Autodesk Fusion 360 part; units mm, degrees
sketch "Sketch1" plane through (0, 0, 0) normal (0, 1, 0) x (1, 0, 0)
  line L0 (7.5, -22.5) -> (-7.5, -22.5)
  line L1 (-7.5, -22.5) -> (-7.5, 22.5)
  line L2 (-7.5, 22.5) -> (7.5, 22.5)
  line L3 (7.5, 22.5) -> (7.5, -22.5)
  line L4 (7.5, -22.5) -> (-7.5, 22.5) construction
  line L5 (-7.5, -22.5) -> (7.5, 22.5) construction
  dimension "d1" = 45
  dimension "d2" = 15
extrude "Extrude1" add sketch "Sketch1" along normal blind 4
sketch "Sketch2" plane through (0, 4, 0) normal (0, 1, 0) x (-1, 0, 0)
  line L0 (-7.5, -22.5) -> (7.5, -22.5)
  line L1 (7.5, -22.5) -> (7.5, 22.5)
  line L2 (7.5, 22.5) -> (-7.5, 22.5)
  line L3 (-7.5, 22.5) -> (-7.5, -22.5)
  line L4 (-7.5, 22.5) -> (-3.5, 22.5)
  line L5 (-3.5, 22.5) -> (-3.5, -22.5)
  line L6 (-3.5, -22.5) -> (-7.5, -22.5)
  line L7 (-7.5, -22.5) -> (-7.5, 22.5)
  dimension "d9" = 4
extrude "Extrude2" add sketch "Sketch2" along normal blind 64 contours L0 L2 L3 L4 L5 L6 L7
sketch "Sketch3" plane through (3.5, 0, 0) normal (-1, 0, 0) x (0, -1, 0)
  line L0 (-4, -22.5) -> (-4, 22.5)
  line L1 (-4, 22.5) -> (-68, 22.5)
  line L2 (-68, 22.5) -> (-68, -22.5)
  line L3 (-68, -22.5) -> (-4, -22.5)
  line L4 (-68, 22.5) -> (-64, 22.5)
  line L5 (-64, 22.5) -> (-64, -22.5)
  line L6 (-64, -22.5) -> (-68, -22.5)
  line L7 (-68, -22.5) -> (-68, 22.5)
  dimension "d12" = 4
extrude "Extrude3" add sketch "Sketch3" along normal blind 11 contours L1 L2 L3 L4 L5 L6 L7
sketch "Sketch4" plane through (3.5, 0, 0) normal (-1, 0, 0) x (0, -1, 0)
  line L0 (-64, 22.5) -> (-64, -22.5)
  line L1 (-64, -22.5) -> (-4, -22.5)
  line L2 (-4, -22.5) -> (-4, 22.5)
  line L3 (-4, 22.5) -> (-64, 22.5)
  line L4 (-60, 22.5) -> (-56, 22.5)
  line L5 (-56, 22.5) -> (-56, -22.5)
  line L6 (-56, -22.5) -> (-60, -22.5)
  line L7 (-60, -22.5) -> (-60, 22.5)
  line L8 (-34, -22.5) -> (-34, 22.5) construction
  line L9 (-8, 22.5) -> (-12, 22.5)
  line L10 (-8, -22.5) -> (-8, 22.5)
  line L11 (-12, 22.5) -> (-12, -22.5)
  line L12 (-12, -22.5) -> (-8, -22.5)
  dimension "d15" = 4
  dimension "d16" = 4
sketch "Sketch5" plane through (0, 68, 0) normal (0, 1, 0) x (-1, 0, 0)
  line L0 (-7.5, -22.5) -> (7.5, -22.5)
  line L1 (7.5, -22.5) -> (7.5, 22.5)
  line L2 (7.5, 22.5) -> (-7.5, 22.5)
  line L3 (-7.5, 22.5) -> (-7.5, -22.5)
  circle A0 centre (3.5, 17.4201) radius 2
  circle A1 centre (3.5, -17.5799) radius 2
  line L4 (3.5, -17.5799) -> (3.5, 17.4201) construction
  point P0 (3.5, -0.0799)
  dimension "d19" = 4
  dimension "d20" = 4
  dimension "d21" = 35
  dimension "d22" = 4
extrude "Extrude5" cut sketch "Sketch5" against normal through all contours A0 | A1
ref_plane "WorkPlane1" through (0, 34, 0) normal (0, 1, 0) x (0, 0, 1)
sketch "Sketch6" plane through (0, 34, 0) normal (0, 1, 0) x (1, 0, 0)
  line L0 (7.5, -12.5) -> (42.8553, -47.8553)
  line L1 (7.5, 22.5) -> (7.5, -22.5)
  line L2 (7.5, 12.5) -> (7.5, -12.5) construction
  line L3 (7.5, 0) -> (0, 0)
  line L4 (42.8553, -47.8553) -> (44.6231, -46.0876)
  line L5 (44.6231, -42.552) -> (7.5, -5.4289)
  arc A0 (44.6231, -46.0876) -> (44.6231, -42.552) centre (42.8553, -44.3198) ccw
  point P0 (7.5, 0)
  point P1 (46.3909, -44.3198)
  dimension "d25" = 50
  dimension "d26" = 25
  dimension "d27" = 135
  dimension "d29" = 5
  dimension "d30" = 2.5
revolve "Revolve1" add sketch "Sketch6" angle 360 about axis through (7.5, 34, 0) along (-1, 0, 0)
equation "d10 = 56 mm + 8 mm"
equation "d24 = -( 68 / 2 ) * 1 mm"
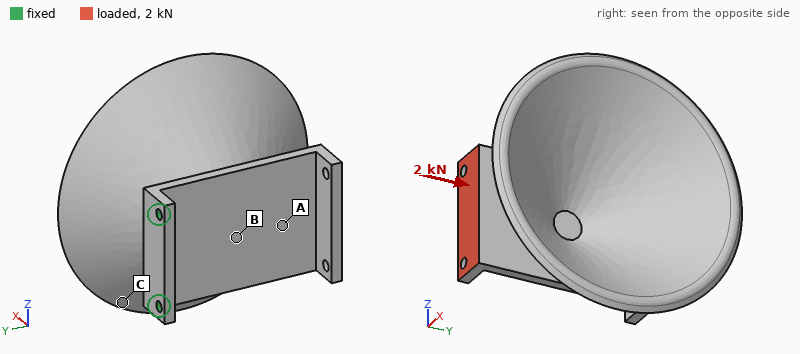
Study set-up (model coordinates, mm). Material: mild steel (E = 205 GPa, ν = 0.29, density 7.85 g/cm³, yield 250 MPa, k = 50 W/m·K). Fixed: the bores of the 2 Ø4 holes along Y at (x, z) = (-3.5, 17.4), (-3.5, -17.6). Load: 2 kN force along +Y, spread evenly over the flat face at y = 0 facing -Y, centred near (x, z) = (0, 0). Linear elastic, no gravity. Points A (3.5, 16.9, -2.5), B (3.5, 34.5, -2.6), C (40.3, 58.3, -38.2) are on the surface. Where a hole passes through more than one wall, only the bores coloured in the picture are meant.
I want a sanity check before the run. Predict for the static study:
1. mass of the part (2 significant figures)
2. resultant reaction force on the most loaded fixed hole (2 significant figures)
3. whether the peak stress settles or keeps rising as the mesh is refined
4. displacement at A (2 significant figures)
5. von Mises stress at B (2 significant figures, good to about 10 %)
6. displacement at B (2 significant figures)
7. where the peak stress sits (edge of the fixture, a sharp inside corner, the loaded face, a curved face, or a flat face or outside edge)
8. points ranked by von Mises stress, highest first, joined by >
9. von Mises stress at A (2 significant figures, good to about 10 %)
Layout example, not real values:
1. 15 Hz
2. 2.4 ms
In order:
1. 480 g
2. 1.0 kN
3. keeps rising
4. 0.20 mm
5. 26 MPa
6. 0.098 mm
7. edge of the fixture
8. A > B > C
9. 98 MPa
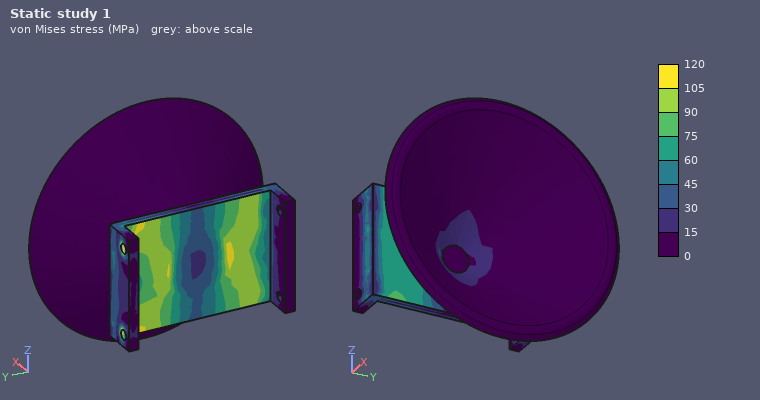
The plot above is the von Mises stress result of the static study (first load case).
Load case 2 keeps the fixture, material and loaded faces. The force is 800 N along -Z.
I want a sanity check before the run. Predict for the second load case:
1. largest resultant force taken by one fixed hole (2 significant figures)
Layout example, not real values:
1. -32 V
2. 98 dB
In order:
1. 1.5 kN
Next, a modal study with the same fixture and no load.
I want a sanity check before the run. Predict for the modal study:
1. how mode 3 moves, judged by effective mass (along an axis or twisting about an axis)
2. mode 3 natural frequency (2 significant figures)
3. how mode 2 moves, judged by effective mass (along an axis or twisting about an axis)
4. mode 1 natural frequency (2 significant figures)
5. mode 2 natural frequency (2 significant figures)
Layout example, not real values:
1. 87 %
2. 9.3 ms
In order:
1. along Z
2. 1300 Hz
3. along Z
4. 220 Hz
5. 540 Hz
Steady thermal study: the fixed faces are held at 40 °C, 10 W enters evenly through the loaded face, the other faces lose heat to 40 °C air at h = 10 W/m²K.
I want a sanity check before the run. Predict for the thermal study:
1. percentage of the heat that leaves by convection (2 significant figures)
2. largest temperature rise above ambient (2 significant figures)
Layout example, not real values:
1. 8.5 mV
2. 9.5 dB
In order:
1. 55 %
2. 54 K
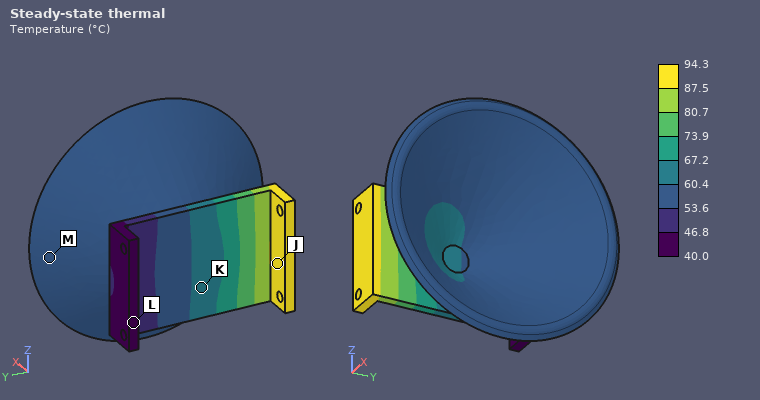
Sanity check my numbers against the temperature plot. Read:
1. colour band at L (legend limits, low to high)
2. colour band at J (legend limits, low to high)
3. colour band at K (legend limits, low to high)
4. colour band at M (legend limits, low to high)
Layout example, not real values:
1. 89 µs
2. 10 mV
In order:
1. 40.0 to 46.8 °C
2. 87.5 to 94.3 °C
3. 60.4 to 67.2 °C
4. 53.6 to 60.4 °C
